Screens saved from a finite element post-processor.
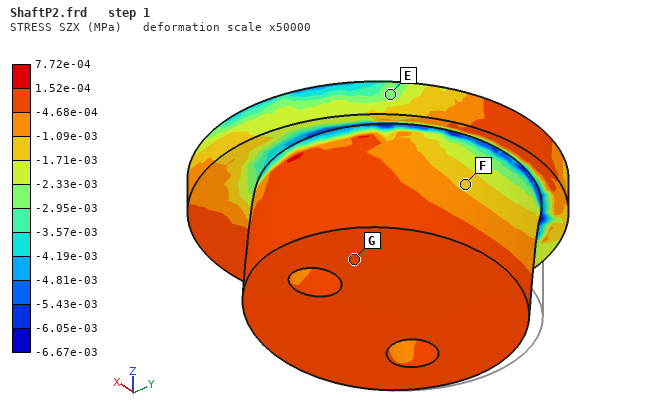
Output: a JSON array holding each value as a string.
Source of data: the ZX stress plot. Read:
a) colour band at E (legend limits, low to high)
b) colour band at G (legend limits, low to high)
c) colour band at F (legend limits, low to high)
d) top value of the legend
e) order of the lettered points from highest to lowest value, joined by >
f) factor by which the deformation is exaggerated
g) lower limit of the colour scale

["-2.95e-03 to -2.33e-03 MPa", "-4.68e-04 to 1.52e-04 MPa", "-1.71e-03 to -1.09e-03 MPa", "7.72e-04 MPa", "G > F > E", "50000", "-6.67e-03 MPa"]
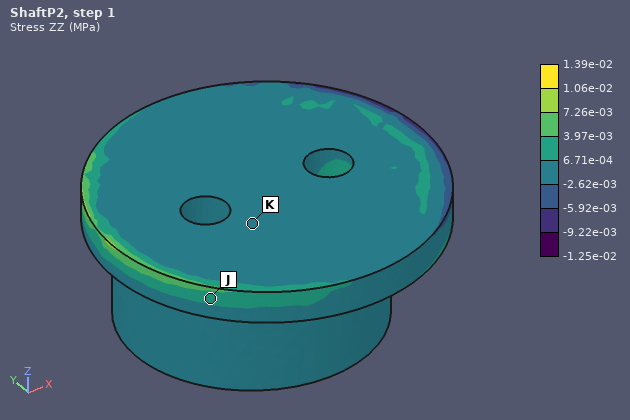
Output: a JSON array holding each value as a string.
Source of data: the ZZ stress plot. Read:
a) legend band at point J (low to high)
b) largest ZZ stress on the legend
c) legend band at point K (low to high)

["6.71e-04 to 3.97e-03 MPa", "1.39e-02 MPa", "-2.62e-03 to 6.71e-04 MPa"]
